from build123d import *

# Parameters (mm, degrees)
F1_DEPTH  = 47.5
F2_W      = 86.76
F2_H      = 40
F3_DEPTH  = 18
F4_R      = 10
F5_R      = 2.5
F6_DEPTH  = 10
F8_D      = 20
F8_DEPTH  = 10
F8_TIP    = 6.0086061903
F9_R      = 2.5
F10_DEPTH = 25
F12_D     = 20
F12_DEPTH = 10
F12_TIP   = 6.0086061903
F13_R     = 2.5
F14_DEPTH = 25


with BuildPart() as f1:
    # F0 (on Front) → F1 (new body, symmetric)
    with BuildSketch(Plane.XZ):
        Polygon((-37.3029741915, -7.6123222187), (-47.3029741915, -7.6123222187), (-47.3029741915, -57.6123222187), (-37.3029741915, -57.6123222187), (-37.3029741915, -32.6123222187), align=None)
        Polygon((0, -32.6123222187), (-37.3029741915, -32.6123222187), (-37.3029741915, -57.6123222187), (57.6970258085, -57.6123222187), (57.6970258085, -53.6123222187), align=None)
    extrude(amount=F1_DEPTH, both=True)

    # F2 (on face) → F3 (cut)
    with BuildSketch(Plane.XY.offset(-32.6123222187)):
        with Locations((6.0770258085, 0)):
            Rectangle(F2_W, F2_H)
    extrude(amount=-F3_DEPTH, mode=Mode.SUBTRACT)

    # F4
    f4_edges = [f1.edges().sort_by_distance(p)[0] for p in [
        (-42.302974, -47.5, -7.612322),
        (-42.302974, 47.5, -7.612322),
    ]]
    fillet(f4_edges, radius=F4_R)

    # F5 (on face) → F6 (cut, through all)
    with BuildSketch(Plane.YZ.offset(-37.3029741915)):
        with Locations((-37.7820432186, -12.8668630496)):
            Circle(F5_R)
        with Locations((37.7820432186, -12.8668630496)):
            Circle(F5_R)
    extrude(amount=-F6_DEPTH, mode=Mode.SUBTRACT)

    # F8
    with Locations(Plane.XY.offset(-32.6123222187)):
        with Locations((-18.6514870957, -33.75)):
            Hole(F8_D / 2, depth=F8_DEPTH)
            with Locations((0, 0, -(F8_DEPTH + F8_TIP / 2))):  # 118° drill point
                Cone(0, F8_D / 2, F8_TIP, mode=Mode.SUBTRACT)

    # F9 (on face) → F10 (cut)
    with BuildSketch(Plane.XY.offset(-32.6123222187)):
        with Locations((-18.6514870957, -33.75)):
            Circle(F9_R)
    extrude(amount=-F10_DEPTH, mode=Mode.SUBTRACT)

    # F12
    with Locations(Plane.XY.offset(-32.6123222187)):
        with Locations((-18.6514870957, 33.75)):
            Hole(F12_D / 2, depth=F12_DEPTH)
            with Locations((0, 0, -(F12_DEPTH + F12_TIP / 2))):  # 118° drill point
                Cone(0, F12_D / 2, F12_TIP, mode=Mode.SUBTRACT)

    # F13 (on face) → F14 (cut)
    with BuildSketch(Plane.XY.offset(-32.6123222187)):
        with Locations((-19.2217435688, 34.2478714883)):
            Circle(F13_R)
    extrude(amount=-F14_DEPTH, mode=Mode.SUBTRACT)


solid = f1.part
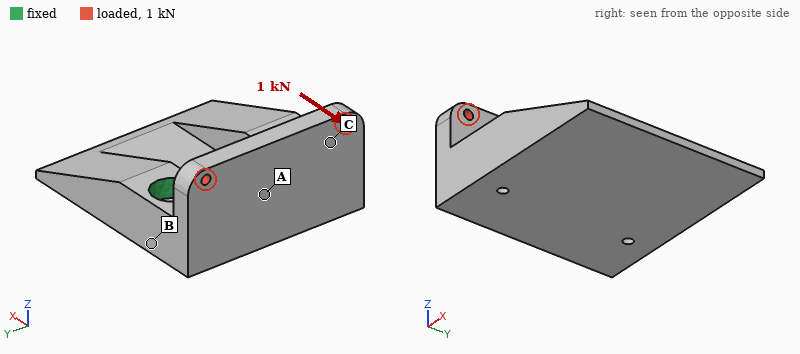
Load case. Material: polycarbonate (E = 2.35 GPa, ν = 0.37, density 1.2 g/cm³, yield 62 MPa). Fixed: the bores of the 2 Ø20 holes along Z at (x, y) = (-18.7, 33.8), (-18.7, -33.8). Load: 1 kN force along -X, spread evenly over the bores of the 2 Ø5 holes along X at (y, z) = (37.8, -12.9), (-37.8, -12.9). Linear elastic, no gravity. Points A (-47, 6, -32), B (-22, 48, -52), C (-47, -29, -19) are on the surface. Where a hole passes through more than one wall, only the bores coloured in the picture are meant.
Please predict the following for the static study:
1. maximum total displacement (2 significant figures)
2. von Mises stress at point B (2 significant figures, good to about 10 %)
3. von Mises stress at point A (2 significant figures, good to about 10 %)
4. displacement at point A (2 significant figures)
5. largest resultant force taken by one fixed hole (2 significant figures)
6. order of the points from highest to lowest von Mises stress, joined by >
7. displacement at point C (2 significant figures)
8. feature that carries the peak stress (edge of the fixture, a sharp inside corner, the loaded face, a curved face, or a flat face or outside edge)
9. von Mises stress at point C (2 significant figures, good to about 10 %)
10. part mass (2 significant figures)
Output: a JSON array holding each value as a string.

["0.69 mm", "2.1 MPa", "5.0 MPa", "0.13 mm", "500 N", "C > A > B", "0.36 mm", "the loaded face", "7.7 MPa", "190 g"]
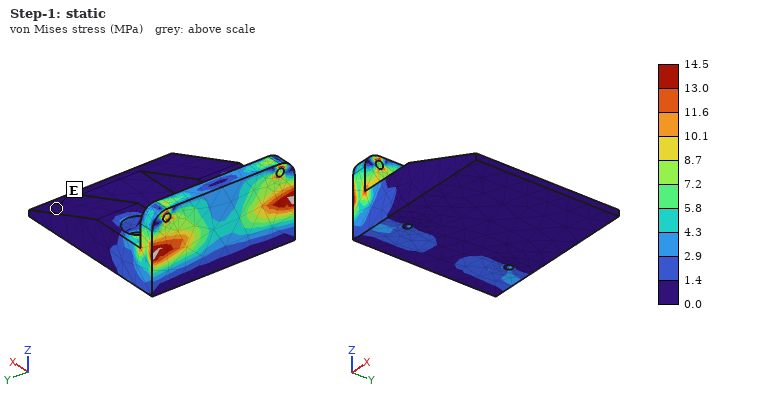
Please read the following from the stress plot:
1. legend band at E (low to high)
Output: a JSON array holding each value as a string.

["0.0 to 1.4 MPa"]
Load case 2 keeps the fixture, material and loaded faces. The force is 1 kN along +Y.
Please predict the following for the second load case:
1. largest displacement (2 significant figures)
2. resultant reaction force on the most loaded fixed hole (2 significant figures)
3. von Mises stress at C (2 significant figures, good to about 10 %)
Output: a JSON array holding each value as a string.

["0.14 mm", "620 N", "2.4 MPa"]
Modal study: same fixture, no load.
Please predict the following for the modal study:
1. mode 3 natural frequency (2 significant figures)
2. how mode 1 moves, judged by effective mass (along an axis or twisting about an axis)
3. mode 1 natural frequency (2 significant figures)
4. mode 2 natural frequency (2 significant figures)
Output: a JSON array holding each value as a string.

["1800 Hz", "along Z", "1000 Hz", "1400 Hz"]
